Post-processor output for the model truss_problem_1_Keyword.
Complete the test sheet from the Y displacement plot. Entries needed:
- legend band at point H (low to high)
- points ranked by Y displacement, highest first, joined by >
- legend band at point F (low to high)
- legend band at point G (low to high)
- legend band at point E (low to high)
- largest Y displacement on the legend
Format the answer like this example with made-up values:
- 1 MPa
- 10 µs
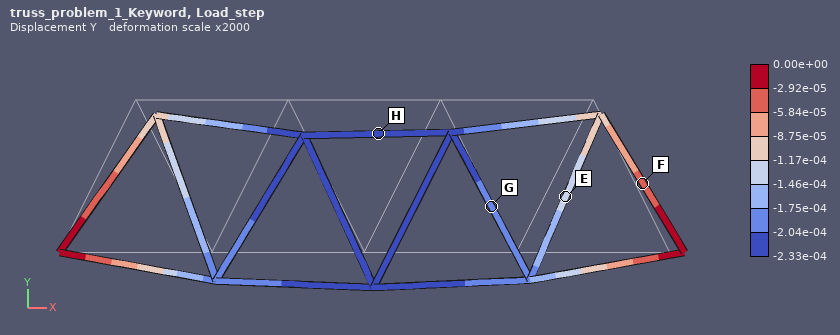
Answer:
- -2.33e-04 to -2.04e-04
- F > E > G > H
- -5.84e-05 to -2.92e-05
- -2.04e-04 to -1.75e-04
- -1.46e-04 to -1.17e-04
- 0.00e+00
